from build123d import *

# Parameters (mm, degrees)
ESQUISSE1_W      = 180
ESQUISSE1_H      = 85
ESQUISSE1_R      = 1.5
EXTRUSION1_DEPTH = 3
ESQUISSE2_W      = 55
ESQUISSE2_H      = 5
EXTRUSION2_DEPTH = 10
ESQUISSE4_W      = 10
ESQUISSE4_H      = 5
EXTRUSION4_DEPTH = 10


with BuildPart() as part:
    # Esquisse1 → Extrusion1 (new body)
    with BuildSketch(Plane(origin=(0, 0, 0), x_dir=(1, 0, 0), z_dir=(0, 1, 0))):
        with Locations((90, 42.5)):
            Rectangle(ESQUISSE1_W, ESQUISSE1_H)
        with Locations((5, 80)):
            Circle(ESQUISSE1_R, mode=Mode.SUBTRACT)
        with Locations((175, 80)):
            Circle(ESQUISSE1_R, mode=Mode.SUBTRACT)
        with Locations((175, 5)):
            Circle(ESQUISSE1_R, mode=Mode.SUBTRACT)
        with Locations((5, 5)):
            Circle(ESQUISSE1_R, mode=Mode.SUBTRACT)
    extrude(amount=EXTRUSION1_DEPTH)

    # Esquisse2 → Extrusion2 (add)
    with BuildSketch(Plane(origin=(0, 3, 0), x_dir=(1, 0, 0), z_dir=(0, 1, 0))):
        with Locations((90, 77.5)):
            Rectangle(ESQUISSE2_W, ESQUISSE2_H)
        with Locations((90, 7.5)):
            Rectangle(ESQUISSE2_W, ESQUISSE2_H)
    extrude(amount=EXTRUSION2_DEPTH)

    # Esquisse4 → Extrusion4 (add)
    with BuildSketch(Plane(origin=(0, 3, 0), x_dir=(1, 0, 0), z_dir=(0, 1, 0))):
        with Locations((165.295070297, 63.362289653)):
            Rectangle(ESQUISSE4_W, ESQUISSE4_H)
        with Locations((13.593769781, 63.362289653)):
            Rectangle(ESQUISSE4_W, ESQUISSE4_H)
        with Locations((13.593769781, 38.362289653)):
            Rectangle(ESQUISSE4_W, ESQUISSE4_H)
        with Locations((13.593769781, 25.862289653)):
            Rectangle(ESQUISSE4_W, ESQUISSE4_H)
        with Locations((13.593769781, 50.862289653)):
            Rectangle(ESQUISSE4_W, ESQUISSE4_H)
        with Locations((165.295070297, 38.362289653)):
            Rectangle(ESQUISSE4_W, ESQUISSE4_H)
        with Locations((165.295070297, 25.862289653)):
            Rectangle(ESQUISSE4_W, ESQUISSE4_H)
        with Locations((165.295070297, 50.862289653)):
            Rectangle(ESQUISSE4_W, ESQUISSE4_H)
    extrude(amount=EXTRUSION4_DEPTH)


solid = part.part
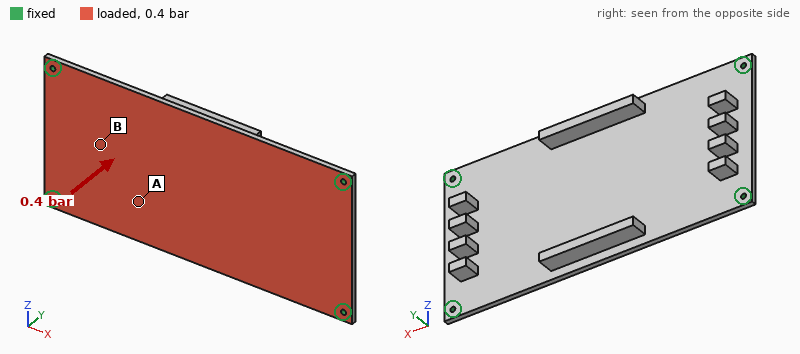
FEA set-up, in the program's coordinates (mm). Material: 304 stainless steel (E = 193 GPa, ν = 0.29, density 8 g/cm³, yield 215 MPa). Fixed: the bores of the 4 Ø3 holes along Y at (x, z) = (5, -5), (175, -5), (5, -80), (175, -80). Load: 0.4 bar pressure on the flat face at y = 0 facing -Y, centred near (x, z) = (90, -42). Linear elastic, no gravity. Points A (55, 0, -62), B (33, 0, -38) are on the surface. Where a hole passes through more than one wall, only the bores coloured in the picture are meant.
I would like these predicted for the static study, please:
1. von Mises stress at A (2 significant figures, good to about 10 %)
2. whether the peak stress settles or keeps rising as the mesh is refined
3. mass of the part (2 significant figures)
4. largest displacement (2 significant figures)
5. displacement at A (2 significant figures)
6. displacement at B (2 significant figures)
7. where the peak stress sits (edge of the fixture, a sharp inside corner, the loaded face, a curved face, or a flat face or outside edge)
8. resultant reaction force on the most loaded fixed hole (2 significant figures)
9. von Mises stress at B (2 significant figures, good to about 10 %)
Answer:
28 MPa
keeps rising
440 g
0.18 mm
0.15 mm
0.096 mm
edge of the fixture
160 N
10.0 MPa
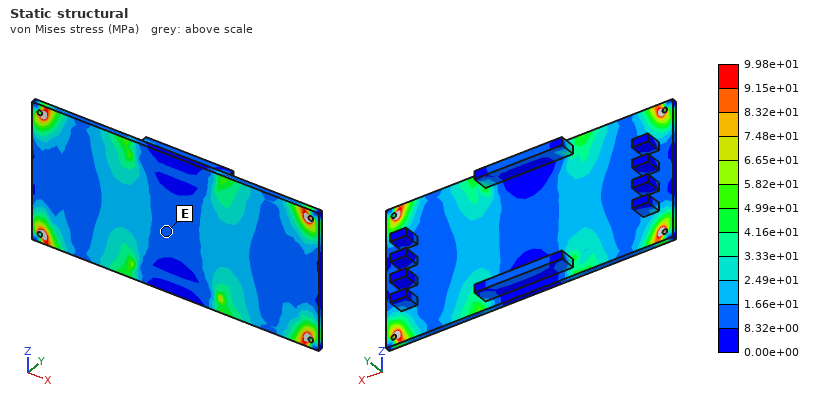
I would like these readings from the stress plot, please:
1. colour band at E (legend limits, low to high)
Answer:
8.32e+00 to 1.66e+01 MPa
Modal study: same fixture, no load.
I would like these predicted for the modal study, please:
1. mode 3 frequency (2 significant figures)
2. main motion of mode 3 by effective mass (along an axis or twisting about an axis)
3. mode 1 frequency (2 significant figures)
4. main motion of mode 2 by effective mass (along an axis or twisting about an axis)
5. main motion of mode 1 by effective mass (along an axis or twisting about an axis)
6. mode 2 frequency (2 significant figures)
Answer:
1200 Hz
twisting about Z
490 Hz
twisting about X
along Y
810 Hz
